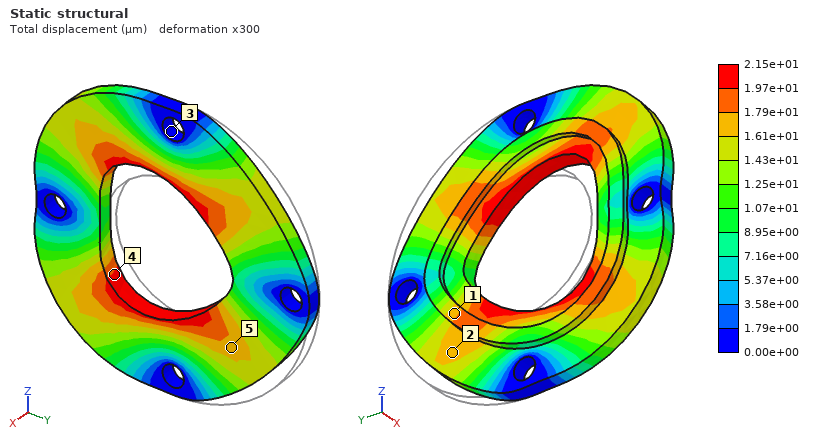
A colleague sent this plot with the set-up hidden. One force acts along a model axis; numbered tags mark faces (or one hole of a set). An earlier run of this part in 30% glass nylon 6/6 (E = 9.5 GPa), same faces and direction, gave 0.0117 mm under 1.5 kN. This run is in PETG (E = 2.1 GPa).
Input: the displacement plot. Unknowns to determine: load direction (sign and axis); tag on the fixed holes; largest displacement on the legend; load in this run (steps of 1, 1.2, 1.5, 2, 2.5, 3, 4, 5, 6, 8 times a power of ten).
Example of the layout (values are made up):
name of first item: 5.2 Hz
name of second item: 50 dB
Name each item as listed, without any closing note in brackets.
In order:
load direction: -Y
tag on the fixed holes: 3
largest displacement on the legend: 2.15e+01 µm
load in this run: 600 N
